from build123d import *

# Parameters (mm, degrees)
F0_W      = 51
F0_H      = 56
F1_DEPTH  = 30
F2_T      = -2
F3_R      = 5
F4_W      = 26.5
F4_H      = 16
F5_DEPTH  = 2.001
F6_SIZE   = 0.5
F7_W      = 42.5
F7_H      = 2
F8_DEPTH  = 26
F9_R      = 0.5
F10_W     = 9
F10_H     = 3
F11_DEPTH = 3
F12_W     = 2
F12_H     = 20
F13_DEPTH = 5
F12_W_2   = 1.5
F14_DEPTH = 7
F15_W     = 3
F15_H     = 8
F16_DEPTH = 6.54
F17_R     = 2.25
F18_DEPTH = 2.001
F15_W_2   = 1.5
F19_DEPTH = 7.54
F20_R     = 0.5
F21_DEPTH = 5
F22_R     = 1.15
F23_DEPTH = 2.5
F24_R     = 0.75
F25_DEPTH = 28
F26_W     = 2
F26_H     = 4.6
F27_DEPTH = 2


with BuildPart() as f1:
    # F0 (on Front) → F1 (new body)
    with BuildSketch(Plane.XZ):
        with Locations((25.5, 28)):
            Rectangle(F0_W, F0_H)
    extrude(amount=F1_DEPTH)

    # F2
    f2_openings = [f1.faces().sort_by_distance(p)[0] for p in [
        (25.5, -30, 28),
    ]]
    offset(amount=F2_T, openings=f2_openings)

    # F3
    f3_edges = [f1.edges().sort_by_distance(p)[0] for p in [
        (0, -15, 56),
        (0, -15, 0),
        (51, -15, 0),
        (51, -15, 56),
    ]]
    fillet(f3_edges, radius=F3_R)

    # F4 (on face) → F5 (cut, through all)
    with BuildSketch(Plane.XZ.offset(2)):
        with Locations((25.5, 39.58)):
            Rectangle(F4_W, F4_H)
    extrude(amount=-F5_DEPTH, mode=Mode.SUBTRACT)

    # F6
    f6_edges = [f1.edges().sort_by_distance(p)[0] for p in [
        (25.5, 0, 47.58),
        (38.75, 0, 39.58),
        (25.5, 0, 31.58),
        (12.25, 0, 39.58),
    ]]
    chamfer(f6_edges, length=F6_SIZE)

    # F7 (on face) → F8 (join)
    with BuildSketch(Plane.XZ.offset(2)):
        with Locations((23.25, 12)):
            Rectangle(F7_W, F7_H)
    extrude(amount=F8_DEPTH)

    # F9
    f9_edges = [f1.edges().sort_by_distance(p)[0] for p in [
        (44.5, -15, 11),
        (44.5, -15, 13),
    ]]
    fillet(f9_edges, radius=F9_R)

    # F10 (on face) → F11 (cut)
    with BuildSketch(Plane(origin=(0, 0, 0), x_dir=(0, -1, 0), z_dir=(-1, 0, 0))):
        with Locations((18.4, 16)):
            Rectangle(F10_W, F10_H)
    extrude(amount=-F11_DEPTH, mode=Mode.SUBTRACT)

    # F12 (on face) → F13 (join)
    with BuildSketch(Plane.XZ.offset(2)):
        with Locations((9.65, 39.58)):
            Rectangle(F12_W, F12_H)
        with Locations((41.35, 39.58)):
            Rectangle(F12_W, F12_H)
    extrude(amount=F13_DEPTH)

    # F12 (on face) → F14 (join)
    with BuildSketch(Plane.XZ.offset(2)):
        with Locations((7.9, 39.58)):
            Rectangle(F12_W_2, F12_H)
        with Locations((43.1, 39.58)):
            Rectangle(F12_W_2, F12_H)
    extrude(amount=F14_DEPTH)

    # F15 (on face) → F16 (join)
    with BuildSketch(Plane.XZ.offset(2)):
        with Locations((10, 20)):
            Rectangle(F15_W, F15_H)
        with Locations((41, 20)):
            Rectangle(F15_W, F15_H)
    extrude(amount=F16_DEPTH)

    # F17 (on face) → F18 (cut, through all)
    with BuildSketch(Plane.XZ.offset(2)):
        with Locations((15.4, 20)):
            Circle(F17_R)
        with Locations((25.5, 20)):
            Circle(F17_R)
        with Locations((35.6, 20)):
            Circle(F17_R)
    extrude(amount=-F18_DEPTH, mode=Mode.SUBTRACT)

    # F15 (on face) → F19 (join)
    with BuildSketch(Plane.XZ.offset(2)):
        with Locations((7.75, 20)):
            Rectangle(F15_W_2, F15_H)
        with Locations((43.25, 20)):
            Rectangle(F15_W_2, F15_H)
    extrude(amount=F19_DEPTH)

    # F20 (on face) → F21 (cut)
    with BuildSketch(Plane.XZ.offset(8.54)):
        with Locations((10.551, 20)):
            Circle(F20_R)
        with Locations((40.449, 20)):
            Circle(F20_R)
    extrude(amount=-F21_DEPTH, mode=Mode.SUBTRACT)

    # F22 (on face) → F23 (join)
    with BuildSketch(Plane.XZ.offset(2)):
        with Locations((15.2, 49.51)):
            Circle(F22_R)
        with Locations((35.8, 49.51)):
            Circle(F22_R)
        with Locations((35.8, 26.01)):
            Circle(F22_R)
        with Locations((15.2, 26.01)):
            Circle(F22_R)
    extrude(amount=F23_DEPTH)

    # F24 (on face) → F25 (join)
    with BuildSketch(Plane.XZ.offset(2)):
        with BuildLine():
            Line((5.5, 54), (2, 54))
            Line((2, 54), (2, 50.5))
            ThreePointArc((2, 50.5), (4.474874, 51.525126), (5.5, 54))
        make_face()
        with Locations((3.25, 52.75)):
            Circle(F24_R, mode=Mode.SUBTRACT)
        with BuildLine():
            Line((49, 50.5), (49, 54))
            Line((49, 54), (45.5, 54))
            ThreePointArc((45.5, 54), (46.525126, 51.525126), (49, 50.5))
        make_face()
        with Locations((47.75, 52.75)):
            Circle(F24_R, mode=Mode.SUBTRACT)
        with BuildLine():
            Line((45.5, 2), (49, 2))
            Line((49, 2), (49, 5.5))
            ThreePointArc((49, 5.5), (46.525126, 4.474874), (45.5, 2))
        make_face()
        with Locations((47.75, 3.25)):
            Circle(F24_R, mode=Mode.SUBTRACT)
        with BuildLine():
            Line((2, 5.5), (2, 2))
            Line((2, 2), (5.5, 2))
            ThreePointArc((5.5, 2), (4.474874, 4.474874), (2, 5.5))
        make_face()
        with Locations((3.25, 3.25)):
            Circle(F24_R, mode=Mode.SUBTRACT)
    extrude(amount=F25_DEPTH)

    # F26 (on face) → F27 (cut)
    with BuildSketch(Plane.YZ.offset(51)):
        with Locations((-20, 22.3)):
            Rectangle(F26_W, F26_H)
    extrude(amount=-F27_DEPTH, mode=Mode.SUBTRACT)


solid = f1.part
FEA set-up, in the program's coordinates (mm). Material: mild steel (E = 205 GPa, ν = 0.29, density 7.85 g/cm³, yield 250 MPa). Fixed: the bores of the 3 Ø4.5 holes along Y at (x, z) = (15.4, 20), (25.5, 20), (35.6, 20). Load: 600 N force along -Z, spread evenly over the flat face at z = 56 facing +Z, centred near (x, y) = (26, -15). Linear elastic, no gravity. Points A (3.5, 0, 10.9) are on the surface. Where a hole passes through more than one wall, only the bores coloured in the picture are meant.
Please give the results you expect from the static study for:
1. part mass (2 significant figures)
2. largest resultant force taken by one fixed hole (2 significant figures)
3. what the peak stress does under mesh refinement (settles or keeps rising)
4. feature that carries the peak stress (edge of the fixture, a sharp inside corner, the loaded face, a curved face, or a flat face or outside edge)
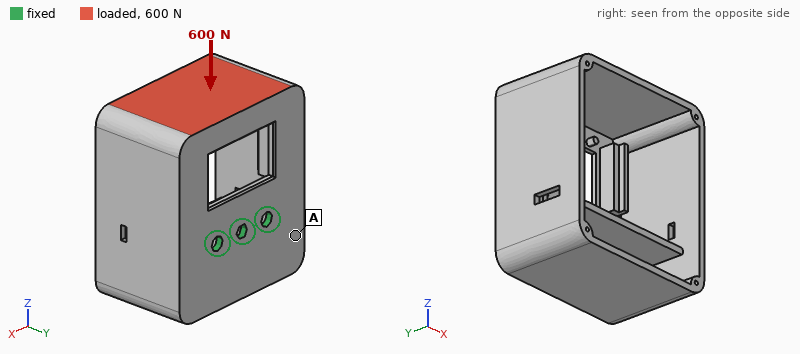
160 g
340 N
keeps rising
edge of the fixture
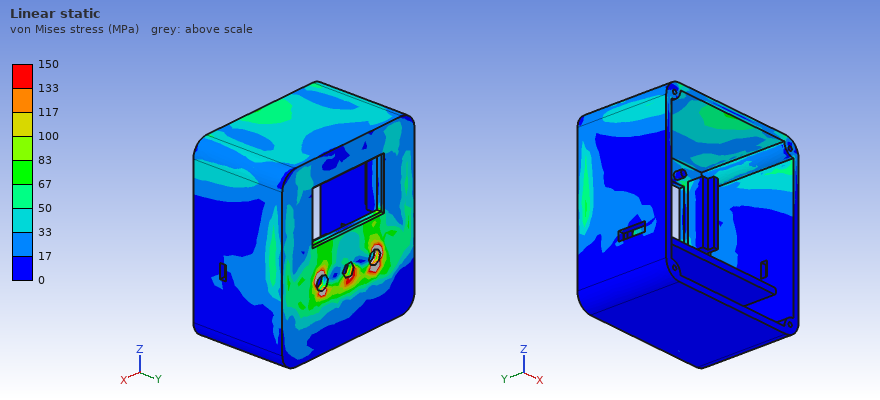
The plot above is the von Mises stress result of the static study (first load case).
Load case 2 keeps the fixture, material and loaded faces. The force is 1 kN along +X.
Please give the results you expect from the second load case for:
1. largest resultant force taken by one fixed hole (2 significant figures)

1.5 kN
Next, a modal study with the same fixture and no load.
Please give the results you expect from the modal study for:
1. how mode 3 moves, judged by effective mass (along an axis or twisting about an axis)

along X
